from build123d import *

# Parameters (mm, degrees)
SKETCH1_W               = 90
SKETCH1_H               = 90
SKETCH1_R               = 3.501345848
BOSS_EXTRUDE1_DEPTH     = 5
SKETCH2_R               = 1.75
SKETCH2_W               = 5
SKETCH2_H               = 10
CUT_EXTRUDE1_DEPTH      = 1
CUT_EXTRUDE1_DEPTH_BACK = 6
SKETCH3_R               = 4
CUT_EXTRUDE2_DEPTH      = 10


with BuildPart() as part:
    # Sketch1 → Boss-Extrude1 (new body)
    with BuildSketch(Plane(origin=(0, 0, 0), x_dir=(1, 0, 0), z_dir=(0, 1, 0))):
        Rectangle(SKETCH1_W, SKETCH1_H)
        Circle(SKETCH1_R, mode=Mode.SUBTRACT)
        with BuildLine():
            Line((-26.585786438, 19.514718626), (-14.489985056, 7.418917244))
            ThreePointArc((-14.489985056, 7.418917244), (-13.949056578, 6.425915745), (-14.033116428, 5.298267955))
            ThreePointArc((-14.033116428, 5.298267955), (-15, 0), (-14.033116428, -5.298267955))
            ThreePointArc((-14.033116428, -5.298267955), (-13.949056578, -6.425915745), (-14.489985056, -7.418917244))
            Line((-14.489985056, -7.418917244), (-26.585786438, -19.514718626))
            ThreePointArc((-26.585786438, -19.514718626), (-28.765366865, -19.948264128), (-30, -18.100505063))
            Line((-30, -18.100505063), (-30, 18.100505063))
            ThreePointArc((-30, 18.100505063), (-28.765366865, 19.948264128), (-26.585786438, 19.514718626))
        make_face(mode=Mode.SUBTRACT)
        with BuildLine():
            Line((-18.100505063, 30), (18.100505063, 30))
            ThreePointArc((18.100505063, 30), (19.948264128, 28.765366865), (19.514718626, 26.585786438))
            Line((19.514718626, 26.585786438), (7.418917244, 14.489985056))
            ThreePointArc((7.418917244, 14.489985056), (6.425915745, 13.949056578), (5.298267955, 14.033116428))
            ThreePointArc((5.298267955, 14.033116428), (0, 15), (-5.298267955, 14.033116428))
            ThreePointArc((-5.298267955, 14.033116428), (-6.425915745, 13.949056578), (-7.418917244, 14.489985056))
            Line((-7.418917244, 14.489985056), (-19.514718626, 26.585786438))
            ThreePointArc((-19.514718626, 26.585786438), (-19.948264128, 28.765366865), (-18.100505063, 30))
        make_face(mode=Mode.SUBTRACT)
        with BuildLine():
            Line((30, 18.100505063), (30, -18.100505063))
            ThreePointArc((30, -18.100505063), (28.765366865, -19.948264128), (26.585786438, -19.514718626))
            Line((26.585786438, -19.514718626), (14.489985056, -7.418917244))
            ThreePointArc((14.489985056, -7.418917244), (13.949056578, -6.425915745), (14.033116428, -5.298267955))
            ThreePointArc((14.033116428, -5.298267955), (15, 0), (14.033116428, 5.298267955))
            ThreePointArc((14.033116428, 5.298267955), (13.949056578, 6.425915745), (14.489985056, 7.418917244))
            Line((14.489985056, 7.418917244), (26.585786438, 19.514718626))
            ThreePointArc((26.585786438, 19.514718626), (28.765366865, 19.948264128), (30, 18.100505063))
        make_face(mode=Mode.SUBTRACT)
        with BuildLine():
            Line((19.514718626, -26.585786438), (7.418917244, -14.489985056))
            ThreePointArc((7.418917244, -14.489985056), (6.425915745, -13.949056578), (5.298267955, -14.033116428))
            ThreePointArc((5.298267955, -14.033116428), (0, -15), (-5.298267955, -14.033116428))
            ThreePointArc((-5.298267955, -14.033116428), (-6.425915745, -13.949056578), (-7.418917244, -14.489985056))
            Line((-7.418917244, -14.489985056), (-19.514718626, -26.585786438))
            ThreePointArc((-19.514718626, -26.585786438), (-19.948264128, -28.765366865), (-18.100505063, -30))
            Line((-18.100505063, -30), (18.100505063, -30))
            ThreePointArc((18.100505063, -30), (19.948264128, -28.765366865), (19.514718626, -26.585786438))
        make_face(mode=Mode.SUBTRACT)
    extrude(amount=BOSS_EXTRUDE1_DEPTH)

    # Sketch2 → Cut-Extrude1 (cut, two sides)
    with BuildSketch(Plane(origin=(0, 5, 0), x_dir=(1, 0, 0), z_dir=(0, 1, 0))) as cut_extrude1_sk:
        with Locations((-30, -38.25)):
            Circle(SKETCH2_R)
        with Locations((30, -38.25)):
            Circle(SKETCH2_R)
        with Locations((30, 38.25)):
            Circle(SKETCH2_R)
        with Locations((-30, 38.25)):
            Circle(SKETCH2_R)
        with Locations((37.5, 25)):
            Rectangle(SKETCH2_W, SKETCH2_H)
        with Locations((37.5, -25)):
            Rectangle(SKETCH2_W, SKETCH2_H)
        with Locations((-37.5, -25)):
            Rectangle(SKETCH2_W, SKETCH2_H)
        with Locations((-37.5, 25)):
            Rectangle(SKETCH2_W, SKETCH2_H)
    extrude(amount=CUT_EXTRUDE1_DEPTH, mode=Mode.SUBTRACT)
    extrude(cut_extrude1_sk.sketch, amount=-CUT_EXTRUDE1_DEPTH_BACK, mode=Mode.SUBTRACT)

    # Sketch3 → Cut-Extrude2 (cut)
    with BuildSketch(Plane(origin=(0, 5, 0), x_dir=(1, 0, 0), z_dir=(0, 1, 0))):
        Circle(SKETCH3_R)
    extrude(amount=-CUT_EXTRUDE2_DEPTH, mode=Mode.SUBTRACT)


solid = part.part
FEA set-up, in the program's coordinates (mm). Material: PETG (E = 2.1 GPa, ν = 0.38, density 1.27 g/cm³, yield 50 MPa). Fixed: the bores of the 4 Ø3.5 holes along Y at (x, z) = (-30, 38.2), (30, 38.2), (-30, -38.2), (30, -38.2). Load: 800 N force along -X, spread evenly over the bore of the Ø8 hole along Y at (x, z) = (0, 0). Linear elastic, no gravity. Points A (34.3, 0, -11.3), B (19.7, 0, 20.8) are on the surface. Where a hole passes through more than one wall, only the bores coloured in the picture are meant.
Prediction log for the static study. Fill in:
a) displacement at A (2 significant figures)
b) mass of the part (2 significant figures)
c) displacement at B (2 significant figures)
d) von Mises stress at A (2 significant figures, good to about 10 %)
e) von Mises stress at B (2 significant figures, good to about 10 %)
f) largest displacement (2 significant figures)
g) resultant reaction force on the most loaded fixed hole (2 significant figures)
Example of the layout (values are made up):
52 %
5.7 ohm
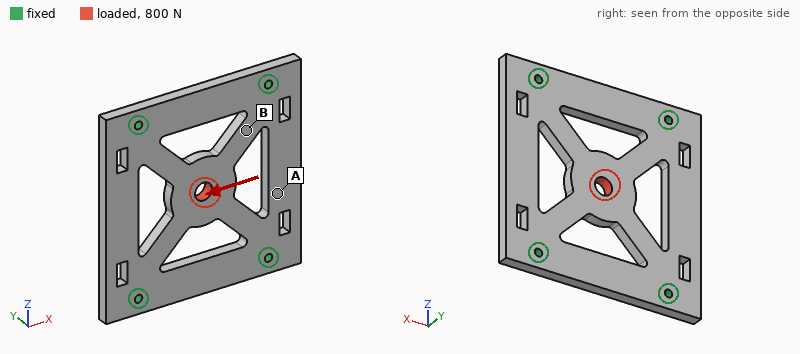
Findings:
0.064 mm
38 g
0.080 mm
0.98 MPa
5.2 MPa
0.18 mm
240 N
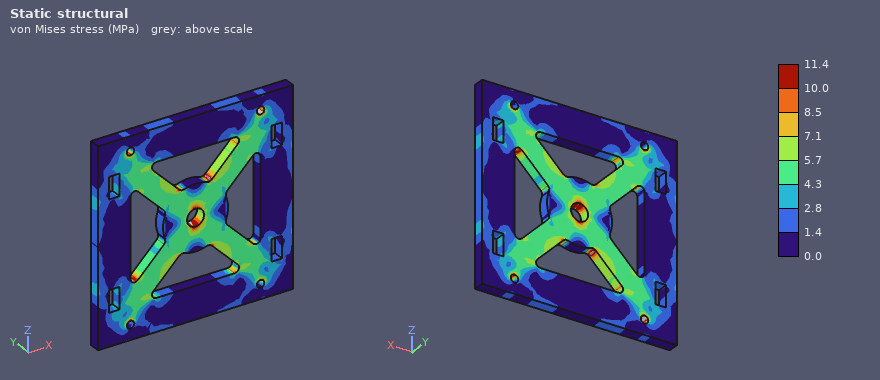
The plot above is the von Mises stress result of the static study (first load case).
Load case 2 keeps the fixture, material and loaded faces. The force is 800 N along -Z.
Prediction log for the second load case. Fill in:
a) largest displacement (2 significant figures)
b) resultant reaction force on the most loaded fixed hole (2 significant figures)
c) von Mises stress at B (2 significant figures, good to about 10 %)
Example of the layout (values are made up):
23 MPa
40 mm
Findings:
0.15 mm
230 N
5.6 MPa
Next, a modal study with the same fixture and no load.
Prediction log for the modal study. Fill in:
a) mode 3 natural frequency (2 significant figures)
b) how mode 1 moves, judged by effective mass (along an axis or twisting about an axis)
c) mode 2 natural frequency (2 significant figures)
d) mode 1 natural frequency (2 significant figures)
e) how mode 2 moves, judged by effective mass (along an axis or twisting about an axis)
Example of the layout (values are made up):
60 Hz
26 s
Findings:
1200 Hz
along Y
1100 Hz
850 Hz
twisting about Z
